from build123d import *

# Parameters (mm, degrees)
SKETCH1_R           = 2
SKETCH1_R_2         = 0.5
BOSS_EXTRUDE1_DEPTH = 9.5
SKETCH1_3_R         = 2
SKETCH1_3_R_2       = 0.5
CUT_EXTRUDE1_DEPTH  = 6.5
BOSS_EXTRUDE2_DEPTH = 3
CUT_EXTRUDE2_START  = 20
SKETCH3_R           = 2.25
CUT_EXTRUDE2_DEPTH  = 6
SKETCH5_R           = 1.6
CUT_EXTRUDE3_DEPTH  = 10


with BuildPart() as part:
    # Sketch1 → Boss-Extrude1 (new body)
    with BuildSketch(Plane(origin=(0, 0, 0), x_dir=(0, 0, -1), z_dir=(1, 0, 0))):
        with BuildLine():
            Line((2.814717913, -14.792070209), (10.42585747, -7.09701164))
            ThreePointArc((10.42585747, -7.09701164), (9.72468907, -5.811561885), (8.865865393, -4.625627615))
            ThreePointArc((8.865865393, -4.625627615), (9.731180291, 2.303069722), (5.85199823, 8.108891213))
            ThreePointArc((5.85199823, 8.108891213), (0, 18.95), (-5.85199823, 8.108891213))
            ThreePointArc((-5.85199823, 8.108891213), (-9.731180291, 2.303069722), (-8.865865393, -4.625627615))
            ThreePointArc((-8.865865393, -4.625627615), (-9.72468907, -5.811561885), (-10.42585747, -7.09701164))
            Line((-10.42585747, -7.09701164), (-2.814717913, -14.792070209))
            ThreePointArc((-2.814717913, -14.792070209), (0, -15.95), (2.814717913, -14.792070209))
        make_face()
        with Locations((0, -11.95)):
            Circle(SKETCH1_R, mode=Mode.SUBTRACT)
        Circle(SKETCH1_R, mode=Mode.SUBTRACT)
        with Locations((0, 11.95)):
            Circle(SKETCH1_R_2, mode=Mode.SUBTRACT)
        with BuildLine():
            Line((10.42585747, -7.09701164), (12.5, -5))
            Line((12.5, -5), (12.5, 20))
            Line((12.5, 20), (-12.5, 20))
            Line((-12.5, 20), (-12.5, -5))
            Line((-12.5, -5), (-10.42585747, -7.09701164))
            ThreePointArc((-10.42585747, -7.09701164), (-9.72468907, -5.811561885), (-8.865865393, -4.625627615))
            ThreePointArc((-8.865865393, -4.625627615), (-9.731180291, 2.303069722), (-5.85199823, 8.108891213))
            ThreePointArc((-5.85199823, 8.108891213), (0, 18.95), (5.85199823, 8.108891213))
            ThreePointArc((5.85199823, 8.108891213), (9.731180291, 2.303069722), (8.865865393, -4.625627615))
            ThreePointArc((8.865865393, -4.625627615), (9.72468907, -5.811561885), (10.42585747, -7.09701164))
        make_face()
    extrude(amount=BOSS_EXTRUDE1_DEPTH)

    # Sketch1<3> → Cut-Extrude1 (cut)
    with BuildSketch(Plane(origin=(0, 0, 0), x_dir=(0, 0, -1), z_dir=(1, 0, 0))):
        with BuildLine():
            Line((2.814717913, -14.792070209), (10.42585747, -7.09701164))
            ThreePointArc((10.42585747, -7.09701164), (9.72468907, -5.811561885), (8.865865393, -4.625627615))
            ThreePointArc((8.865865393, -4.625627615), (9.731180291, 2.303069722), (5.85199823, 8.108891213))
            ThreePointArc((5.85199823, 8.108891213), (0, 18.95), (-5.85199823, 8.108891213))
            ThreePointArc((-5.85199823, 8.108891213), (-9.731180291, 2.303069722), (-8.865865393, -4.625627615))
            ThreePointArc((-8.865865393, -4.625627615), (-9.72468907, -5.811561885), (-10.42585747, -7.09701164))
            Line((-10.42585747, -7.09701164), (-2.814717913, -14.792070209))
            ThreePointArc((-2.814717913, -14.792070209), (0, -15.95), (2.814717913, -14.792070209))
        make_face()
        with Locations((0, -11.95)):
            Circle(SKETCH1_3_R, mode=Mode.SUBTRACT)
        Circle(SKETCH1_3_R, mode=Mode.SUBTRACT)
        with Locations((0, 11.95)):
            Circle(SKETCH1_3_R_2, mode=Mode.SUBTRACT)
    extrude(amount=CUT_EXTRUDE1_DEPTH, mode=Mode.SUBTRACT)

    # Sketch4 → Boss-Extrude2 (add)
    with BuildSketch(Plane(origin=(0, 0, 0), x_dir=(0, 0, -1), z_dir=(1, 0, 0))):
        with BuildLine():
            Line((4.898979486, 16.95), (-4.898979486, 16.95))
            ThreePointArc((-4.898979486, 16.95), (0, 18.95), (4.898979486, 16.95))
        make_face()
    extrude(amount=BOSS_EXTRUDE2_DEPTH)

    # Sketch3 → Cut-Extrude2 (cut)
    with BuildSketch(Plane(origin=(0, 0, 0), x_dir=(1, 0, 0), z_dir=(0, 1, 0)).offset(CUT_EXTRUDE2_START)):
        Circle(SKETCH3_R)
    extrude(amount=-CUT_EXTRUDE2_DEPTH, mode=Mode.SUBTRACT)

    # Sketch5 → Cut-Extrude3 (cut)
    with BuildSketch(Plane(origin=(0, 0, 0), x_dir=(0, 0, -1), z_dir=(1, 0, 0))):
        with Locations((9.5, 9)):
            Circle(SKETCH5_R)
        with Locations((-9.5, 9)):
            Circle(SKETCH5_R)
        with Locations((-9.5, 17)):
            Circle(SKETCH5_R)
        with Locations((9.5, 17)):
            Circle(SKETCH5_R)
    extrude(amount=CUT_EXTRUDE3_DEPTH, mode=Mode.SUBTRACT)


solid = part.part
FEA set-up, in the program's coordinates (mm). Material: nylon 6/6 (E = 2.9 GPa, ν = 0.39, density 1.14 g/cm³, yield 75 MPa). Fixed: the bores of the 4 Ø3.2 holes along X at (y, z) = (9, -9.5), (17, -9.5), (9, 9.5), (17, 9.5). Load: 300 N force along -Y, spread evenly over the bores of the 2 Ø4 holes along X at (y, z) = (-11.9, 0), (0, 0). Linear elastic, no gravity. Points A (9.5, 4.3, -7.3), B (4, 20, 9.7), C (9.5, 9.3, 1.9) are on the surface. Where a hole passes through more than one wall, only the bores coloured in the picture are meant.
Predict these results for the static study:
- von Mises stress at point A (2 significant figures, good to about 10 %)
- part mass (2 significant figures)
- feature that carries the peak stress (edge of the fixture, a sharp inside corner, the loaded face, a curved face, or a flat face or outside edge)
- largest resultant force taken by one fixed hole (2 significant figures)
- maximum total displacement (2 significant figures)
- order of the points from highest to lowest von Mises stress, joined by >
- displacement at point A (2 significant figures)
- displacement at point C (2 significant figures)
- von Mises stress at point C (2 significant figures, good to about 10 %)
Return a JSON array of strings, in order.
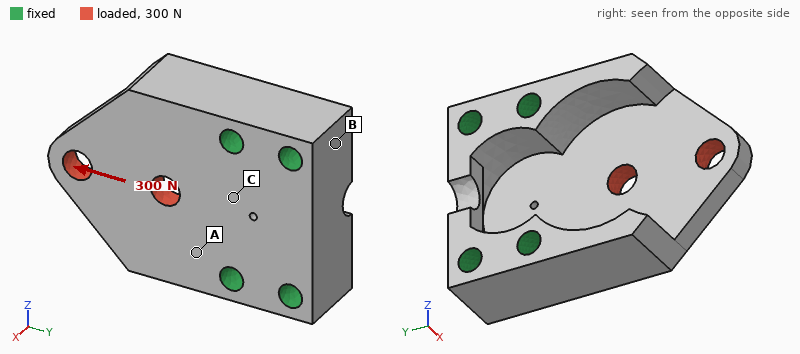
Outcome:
["5.7 MPa", "4.2 g", "the loaded face", "130 N", "58 µm", "A > C > B", "9.9 µm", "9.5 µm", "2.6 MPa"]
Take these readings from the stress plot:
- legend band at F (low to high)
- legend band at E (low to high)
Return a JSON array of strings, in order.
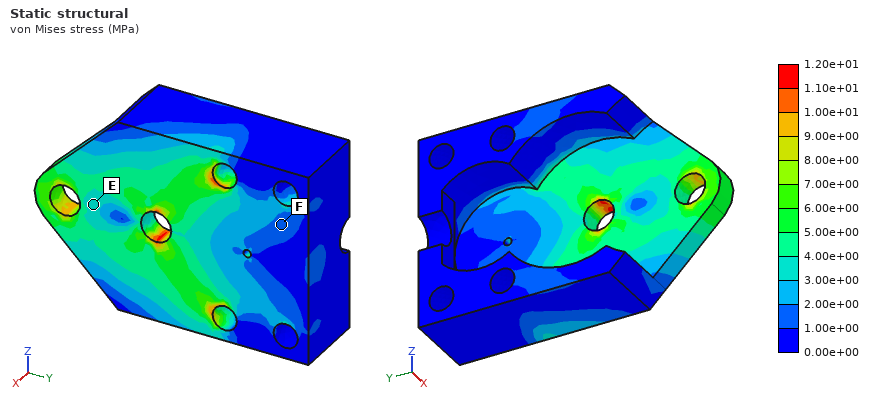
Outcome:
["1.00e+00 to 2.00e+00 MPa", "3.00e+00 to 4.00e+00 MPa"]
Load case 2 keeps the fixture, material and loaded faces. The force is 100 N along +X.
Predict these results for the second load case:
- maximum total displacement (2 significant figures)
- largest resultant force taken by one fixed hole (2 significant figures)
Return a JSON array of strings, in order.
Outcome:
["0.53 mm", "61 N"]
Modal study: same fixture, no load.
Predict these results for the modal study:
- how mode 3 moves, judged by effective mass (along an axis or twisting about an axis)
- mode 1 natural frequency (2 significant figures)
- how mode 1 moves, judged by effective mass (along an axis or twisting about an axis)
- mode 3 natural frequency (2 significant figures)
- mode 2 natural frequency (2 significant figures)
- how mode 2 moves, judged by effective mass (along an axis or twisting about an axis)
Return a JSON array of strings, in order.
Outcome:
["along Z", "3700 Hz", "along X", "9300 Hz", "7700 Hz", "along Z"]
